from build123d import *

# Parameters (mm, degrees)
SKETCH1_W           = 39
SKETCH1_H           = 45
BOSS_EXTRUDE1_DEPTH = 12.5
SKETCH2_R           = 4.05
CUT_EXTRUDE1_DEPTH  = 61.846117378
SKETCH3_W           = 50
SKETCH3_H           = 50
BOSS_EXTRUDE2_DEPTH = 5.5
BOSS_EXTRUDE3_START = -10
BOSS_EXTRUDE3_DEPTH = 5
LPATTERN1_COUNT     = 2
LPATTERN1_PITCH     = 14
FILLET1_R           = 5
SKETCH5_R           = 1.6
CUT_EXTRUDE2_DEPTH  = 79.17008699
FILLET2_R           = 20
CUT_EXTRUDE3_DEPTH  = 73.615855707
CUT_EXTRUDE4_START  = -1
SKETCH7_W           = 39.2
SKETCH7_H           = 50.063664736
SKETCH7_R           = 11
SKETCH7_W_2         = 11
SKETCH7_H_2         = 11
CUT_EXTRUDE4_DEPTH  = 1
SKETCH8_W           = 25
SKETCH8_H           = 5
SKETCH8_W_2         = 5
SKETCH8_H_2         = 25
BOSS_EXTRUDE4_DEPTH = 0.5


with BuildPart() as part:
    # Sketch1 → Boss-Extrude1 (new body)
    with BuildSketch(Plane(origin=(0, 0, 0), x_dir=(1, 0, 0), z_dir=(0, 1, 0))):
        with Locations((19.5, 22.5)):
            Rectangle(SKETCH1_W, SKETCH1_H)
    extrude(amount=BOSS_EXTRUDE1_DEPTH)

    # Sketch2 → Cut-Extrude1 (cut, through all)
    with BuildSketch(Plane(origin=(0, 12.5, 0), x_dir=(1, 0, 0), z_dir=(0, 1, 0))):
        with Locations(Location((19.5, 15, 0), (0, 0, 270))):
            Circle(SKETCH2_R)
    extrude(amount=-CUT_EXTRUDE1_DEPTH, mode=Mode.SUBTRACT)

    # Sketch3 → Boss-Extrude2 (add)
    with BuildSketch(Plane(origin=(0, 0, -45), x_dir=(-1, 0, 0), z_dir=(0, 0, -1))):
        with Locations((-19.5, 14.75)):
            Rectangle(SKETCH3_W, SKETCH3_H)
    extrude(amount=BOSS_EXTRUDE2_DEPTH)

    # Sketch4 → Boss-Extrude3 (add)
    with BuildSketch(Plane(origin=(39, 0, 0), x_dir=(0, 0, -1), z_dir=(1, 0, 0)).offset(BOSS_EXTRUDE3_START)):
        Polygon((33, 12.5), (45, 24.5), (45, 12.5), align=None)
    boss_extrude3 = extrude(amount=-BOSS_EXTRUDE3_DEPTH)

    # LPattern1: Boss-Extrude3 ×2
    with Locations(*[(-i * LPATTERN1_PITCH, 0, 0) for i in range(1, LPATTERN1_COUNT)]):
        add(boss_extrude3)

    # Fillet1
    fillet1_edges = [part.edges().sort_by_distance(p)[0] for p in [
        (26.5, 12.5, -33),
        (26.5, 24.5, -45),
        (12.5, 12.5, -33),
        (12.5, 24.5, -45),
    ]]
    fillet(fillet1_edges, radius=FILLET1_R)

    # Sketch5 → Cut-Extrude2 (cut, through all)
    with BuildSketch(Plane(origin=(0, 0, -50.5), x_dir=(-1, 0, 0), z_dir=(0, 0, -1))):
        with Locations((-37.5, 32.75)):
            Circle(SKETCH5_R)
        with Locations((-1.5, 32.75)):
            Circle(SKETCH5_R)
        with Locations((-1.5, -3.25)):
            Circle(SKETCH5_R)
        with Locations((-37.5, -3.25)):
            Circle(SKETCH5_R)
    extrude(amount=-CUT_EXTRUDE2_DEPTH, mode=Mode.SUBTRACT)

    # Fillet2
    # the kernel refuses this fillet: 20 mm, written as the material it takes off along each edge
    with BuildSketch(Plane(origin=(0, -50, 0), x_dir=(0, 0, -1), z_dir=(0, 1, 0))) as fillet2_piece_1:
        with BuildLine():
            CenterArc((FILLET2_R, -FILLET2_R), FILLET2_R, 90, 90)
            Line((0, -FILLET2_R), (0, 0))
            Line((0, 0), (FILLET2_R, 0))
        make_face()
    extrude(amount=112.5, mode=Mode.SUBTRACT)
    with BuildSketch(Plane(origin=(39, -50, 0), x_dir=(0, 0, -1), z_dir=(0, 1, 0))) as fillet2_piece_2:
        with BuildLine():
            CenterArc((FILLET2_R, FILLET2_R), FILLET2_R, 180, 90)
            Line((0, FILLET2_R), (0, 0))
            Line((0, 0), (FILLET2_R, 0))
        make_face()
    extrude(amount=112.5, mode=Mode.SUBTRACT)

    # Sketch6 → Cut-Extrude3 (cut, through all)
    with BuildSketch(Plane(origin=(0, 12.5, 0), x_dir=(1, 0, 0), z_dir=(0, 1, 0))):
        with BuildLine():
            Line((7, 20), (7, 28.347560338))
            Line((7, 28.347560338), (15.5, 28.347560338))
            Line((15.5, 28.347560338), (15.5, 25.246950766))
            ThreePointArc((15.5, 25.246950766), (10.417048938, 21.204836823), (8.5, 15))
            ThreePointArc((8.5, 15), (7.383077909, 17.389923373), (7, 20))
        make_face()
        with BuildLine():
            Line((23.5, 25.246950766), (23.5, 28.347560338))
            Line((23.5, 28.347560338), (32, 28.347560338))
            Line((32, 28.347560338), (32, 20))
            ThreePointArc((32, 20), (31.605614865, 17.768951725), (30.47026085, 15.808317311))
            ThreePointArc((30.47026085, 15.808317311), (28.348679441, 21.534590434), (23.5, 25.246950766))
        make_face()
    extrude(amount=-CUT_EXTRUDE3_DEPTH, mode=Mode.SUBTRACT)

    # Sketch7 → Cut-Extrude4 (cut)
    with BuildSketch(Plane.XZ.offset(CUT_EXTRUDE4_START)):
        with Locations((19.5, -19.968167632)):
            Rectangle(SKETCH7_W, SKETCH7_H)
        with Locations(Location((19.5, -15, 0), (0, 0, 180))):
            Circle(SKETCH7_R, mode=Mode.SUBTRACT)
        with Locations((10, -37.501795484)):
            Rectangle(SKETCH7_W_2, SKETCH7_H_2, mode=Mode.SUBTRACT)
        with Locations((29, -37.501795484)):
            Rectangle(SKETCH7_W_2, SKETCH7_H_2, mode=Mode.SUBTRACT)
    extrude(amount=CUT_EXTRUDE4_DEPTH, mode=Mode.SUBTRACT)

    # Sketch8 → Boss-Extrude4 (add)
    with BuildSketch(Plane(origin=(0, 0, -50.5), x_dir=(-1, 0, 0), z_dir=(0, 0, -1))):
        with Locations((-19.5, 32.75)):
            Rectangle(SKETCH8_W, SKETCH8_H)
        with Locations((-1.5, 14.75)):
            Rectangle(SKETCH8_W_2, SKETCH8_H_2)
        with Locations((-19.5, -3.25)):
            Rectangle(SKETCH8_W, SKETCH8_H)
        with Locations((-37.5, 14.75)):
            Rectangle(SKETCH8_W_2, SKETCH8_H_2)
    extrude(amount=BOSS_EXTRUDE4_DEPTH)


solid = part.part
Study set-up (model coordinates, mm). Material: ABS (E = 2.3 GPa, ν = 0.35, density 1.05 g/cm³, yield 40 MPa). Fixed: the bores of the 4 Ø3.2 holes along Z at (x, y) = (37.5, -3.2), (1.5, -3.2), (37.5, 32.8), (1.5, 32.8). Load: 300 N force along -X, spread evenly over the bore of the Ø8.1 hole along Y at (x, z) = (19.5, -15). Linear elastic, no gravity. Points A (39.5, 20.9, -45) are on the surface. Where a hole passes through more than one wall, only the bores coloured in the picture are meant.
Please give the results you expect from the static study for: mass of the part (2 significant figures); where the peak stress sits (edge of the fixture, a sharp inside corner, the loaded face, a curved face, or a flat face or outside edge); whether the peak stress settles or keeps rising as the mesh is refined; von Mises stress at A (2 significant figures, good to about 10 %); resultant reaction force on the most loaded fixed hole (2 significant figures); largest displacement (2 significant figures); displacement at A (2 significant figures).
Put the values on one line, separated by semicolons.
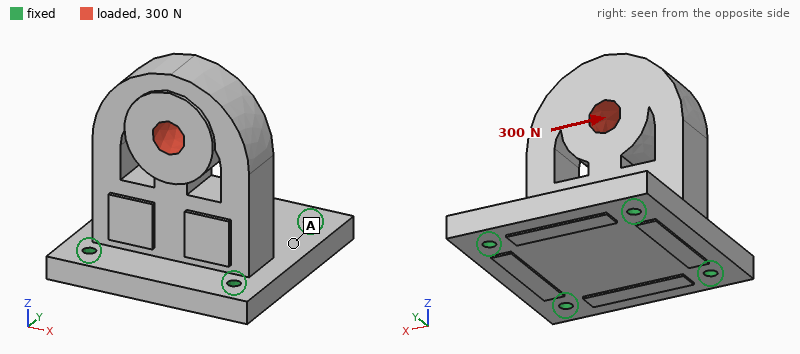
33 g; edge of the fixture; keeps rising; 1.8 MPa; 260 N; 0.24 mm; 0.041 mm
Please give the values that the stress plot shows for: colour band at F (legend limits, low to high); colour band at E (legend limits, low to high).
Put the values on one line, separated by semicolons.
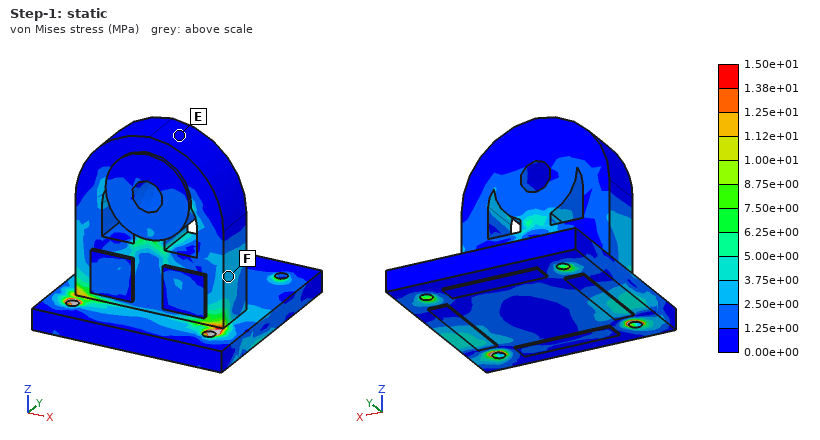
2.50e+00 to 3.75e+00 MPa; 0.00e+00 to 1.25e+00 MPa
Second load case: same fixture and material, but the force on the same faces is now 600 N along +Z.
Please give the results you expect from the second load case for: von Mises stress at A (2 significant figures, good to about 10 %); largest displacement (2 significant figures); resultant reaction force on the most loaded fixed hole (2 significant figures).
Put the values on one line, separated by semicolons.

1.5 MPa; 0.10 mm; 240 N
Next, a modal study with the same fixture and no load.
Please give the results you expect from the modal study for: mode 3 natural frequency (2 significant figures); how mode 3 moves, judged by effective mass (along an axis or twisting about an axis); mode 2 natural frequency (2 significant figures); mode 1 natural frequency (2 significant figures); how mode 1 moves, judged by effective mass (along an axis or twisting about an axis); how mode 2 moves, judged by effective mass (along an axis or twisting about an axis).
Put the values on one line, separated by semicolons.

3000 Hz; along Z; 1900 Hz; 1200 Hz; along Y; along X
